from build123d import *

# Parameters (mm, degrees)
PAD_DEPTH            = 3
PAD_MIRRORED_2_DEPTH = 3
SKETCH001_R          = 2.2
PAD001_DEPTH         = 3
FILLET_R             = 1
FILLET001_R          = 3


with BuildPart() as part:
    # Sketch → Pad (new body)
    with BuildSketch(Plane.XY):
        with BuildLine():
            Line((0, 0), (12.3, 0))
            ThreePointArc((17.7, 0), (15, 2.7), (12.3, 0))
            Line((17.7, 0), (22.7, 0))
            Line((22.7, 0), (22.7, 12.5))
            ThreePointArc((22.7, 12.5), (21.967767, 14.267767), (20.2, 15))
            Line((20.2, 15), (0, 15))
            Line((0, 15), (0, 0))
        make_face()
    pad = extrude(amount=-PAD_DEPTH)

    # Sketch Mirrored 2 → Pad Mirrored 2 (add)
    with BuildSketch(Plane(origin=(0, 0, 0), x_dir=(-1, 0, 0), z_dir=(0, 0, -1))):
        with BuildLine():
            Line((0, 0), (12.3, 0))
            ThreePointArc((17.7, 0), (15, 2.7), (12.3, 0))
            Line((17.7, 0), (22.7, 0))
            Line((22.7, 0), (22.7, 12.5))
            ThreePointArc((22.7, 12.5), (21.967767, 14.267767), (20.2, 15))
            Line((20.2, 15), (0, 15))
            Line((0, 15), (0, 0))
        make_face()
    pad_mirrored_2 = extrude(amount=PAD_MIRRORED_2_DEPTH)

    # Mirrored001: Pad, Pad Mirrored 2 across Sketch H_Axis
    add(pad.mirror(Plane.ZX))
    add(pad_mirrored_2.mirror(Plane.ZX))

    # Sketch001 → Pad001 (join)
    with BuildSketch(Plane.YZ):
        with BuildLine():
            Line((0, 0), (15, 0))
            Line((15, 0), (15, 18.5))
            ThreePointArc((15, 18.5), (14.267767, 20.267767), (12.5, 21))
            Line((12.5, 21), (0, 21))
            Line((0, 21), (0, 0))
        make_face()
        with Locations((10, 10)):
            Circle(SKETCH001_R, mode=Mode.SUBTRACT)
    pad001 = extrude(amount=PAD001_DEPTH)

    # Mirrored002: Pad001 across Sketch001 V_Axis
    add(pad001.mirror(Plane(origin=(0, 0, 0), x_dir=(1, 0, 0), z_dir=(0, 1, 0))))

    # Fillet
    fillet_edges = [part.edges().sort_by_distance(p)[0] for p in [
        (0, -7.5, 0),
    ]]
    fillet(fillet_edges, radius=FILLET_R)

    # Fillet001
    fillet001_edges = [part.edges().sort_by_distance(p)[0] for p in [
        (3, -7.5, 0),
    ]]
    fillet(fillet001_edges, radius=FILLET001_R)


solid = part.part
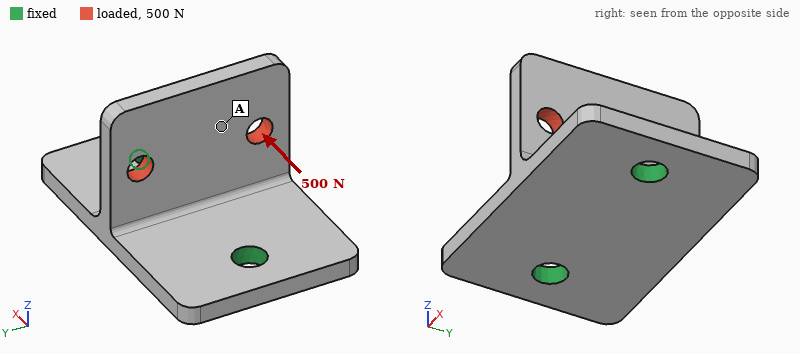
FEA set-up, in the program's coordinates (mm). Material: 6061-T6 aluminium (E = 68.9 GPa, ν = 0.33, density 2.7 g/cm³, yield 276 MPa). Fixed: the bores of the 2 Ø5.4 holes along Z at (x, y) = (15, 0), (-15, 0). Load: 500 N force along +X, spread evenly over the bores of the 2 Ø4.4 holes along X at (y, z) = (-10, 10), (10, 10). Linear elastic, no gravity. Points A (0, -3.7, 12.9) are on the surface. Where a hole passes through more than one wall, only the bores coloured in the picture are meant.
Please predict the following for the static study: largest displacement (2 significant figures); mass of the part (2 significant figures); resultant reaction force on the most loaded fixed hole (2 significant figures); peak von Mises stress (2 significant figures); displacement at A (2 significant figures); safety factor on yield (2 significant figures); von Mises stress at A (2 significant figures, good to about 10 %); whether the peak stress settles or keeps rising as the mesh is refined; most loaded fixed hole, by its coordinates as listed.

0.13 mm
16 g
400 N
97 MPa
0.070 mm
2.9
12 MPa
settles
(15, 0)
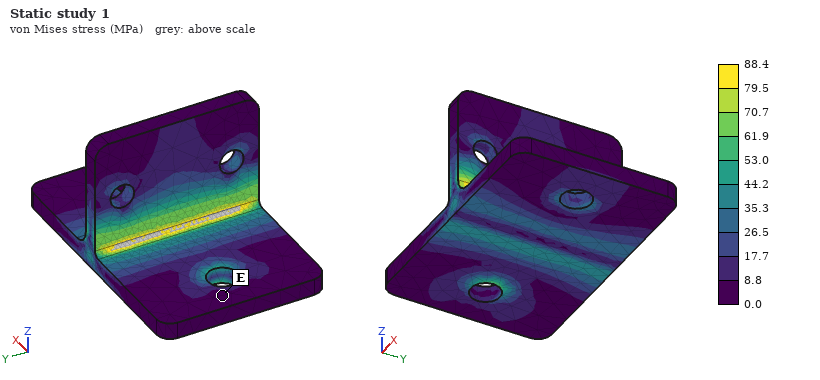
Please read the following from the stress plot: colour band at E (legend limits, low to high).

0.0 to 8.8 MPa
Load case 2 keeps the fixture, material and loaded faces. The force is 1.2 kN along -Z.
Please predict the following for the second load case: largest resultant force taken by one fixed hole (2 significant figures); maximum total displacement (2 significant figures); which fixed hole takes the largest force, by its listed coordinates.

700 N
46 µm
(15, 0)
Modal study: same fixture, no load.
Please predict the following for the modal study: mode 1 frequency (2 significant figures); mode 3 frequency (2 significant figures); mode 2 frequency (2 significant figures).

4900 Hz
9300 Hz
5000 Hz
